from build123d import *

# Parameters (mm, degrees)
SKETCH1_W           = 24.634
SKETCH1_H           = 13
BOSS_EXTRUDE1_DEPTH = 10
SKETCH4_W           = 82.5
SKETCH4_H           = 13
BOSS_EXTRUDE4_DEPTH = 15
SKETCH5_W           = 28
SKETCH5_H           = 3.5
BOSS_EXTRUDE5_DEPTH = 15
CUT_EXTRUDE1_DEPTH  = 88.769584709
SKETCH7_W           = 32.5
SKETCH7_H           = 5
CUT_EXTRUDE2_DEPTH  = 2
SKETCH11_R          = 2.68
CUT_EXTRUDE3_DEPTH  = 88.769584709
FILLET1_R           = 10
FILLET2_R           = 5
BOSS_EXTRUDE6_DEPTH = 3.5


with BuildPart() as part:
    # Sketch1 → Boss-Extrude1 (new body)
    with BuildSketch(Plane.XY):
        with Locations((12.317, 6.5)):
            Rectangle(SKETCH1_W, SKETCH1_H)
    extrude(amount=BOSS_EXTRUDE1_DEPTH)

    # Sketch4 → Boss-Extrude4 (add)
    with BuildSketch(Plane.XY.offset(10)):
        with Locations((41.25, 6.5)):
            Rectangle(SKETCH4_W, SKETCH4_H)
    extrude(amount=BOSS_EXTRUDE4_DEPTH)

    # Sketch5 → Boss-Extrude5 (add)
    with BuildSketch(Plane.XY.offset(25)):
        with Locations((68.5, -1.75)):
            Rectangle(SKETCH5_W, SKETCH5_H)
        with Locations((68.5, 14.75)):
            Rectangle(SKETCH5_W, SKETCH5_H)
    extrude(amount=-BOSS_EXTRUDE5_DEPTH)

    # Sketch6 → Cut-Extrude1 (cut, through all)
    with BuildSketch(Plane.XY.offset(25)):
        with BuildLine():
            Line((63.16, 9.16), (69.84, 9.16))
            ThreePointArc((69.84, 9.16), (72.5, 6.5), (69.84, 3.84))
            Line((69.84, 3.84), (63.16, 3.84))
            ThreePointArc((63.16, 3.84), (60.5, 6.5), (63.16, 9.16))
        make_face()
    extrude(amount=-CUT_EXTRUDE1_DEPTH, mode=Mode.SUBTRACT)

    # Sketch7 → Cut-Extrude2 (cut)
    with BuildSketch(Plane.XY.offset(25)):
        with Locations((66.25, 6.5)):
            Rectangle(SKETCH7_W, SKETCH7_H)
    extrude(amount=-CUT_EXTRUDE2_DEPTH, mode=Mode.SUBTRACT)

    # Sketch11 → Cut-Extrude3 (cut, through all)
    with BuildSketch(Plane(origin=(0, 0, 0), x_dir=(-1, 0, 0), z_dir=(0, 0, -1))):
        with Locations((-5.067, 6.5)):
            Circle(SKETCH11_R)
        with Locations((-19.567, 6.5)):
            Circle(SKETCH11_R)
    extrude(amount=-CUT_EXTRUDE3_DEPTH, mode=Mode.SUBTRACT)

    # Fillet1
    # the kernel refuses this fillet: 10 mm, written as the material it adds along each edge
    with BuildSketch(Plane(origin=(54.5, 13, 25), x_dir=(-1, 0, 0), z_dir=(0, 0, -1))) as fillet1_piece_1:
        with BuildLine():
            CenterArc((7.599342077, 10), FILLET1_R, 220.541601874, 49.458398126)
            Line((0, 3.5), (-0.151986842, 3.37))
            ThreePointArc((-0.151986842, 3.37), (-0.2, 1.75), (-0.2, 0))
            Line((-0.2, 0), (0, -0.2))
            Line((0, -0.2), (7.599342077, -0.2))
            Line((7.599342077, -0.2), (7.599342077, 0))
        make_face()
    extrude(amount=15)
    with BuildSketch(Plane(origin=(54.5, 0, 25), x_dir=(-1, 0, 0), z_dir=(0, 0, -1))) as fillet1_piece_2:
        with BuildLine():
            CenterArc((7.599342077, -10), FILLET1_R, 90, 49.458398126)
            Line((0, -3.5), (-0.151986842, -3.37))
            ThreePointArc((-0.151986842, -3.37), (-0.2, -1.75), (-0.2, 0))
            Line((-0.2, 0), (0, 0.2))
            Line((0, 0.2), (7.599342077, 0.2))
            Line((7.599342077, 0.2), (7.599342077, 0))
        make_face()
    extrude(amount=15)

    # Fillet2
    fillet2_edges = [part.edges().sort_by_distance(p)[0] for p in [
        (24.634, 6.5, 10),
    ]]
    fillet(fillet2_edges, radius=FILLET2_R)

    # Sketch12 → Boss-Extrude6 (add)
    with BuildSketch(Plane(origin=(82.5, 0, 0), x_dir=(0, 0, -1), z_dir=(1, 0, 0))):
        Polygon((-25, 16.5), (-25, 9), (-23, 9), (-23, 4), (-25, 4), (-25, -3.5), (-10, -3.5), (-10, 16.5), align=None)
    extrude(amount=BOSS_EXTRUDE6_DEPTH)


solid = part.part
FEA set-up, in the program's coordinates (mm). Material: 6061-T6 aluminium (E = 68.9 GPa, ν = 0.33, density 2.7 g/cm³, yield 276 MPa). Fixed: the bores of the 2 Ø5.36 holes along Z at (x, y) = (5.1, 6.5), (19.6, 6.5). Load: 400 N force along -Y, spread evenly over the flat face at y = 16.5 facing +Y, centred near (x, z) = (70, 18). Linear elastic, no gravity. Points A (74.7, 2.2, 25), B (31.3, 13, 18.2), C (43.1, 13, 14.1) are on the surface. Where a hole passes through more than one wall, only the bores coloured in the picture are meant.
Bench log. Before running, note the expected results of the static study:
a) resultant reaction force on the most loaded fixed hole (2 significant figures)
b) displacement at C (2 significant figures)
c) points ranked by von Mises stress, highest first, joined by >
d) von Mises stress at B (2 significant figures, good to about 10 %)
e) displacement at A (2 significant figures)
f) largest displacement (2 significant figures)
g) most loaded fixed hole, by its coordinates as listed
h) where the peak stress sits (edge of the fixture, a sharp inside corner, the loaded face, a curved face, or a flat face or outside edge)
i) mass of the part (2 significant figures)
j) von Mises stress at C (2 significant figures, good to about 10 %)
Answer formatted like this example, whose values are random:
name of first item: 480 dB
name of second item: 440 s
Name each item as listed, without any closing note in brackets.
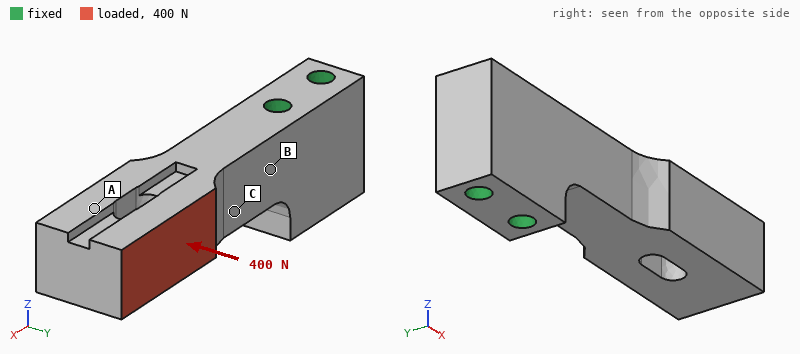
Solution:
resultant reaction force on the most loaded fixed hole: 840 N
displacement at C: 0.032 mm
points ranked by von Mises stress, highest first, joined by >: B > C > A
von Mises stress at B: 35 MPa
displacement at A: 0.11 mm
largest displacement: 0.14 mm
most loaded fixed hole, by its coordinates as listed: (19.6, 6.5)
where the peak stress sits: a curved face
mass of the part: 58 g
von Mises stress at C: 27 MPa
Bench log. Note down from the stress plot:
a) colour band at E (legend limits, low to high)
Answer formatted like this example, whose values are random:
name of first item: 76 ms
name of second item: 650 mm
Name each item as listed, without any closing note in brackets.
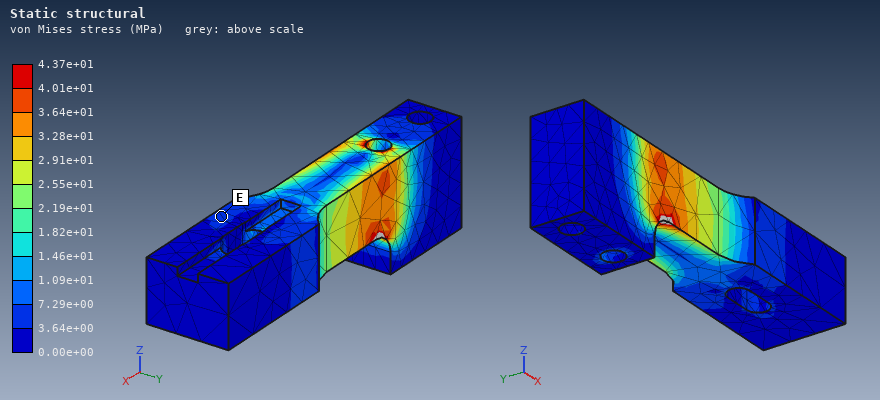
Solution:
colour band at E: 3.64e+00 to 7.29e+00 MPa
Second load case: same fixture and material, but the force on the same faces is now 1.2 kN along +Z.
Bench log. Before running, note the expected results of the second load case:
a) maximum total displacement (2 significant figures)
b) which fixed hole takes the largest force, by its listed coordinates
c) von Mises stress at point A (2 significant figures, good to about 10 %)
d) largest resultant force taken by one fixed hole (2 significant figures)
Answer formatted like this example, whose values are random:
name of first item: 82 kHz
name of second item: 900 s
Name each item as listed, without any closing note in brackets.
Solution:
maximum total displacement: 0.31 mm
which fixed hole takes the largest force, by its listed coordinates: (19.6, 6.5)
von Mises stress at point A: 9.8 MPa
largest resultant force taken by one fixed hole: 1.3 kN
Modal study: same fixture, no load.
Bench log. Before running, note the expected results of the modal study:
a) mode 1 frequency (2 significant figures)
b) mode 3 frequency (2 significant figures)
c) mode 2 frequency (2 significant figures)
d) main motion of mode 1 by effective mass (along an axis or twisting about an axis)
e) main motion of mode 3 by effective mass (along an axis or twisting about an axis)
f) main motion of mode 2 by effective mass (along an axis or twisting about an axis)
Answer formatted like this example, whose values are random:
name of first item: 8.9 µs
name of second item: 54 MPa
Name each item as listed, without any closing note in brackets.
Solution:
mode 1 frequency: 2000 Hz
mode 3 frequency: 8000 Hz
mode 2 frequency: 2500 Hz
main motion of mode 1 by effective mass: along Y
main motion of mode 3 by effective mass: twisting about X
main motion of mode 2 by effective mass: along Z
